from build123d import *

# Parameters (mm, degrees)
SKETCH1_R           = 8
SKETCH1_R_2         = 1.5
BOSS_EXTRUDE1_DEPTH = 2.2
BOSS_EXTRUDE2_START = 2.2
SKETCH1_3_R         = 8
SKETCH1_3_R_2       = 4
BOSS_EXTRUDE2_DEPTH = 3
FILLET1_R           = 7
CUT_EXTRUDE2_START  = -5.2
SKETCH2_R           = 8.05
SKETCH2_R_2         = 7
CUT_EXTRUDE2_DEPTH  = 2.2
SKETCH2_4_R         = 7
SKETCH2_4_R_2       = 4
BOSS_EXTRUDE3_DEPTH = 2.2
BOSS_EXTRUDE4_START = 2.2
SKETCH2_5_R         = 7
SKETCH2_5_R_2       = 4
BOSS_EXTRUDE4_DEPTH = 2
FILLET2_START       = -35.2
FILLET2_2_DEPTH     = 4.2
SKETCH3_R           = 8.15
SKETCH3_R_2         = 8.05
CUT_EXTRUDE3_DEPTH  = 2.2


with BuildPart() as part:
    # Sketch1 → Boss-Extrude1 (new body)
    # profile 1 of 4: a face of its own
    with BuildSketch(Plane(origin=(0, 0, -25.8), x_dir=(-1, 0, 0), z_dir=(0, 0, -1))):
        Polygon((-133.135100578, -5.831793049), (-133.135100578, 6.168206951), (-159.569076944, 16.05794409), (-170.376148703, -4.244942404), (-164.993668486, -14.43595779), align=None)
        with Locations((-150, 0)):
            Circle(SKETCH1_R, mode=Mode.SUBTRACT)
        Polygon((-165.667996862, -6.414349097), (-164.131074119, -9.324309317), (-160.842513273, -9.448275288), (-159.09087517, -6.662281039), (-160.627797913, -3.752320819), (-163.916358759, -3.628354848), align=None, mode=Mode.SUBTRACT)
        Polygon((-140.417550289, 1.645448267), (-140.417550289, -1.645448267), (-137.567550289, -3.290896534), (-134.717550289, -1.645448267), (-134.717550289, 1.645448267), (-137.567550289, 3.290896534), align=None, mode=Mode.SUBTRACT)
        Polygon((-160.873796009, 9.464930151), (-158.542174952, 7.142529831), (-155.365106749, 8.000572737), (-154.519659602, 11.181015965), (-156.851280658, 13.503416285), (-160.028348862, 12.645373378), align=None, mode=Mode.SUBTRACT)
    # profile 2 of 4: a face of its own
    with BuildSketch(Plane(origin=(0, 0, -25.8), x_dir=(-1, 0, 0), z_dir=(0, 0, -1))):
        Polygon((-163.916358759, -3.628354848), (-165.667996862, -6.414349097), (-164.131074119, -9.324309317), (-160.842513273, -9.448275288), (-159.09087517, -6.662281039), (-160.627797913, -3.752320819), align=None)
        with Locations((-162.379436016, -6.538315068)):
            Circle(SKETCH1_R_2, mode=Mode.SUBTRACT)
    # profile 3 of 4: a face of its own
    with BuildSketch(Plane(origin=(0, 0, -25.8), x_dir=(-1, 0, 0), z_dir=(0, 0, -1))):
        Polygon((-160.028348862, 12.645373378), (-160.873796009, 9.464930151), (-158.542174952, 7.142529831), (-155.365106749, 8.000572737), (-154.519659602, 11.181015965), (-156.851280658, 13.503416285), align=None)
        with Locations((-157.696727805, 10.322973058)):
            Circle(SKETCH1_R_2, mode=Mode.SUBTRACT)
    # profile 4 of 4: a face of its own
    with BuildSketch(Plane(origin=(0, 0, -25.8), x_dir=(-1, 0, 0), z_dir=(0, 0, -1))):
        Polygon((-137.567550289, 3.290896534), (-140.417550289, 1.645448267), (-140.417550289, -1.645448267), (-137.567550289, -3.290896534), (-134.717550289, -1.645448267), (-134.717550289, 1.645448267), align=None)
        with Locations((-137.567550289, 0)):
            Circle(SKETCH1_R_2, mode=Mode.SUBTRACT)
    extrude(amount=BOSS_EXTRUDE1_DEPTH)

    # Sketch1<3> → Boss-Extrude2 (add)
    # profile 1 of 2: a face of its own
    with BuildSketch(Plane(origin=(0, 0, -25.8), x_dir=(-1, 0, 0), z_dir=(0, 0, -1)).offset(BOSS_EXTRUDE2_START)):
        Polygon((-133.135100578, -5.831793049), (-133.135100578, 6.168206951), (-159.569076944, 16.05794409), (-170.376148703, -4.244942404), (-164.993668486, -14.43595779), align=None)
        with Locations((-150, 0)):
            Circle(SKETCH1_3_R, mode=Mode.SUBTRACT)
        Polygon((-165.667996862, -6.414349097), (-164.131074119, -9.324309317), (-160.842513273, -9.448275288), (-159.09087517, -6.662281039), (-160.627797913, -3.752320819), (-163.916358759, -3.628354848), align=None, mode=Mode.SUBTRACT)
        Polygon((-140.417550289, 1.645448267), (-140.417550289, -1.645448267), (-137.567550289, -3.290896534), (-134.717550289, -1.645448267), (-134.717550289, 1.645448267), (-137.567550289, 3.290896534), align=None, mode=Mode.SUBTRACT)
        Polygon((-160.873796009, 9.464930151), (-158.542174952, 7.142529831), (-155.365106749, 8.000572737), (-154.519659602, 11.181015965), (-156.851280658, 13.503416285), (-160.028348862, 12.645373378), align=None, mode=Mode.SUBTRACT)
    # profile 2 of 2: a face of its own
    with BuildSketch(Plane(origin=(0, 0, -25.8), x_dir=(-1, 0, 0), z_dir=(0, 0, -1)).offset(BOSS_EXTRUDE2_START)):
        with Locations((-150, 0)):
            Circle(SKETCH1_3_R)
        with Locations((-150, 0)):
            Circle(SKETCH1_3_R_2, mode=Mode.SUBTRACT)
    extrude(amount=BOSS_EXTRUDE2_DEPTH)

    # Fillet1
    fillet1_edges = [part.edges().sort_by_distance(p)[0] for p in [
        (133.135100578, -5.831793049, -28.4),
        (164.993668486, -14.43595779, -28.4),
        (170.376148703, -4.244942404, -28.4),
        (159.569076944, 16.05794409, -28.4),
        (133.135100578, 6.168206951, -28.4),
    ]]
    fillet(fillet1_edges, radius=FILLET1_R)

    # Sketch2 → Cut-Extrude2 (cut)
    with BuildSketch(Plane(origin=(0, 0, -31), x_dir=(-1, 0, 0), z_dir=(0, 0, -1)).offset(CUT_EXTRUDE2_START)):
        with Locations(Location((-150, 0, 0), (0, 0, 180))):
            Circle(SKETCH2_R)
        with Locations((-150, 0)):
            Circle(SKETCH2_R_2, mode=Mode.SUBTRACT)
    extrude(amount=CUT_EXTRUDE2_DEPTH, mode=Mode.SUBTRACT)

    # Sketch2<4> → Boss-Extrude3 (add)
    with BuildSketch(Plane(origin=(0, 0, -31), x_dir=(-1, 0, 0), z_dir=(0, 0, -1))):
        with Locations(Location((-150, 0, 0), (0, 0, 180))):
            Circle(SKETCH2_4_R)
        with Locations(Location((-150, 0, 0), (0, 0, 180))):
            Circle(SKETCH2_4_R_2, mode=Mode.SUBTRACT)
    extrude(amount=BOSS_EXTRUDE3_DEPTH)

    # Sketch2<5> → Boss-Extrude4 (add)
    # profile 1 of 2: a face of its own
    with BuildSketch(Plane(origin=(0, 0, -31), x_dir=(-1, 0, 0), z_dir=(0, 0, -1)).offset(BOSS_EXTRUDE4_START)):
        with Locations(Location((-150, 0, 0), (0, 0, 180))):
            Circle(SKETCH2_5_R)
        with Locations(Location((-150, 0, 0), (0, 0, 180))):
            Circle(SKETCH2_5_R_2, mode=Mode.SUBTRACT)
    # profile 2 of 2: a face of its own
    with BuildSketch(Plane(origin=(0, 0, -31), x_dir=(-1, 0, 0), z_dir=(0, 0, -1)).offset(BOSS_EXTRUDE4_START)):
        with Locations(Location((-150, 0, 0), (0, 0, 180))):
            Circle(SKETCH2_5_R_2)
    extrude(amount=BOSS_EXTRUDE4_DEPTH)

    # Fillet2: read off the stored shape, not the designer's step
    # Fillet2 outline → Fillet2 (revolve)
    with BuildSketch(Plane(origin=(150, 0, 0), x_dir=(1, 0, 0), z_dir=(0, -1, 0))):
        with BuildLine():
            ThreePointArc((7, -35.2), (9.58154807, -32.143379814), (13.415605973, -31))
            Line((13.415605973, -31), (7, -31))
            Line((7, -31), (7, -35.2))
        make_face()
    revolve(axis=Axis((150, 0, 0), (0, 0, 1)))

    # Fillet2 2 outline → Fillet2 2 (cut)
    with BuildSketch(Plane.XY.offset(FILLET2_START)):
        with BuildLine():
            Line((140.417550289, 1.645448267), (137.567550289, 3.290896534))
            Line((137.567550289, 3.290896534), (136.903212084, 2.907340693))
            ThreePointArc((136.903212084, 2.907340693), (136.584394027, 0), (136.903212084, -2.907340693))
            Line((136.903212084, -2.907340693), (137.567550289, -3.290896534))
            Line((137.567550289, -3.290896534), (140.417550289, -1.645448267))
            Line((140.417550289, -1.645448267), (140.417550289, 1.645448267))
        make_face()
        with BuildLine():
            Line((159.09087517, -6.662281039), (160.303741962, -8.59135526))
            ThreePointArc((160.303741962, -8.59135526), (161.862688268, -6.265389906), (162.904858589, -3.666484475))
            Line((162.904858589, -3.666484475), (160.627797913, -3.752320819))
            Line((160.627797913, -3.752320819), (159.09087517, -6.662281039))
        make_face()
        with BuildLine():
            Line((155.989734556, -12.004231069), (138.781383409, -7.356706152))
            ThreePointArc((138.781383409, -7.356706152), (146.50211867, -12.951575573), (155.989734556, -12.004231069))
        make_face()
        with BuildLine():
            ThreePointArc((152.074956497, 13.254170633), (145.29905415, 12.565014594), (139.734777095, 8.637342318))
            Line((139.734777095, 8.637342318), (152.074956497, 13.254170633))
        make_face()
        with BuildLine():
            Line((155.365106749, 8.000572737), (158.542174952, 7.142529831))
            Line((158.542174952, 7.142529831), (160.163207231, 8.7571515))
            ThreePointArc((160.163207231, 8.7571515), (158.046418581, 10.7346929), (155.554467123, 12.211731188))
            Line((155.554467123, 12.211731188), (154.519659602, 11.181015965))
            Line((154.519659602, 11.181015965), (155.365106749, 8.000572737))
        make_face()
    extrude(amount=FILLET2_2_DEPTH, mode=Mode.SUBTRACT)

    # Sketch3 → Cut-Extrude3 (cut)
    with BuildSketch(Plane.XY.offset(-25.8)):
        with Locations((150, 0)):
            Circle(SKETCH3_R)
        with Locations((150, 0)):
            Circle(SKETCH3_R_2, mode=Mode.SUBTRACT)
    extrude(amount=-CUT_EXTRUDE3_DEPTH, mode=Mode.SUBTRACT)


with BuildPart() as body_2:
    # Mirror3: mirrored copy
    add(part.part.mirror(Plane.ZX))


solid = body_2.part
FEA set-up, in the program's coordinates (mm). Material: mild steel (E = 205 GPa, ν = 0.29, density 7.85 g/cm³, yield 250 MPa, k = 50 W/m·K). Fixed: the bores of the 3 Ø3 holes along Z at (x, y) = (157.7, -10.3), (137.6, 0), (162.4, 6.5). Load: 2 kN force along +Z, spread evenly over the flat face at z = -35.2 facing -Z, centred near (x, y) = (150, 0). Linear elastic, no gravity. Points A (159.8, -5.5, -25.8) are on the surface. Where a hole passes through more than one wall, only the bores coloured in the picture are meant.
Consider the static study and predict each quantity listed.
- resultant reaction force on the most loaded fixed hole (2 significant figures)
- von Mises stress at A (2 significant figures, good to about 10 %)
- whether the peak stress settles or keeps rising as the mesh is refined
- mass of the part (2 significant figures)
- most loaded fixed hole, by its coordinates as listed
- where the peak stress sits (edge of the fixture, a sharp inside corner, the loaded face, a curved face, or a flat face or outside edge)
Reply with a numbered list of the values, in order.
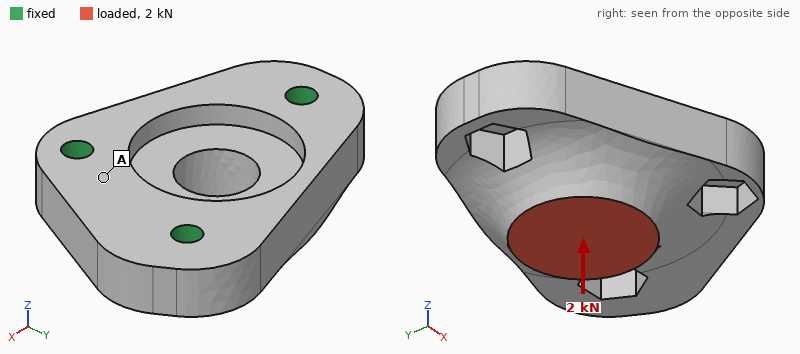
1. 1.1 kN
2. 16 MPa
3. keeps rising
4. 29 g
5. (137.6, 0)
6. edge of the fixture
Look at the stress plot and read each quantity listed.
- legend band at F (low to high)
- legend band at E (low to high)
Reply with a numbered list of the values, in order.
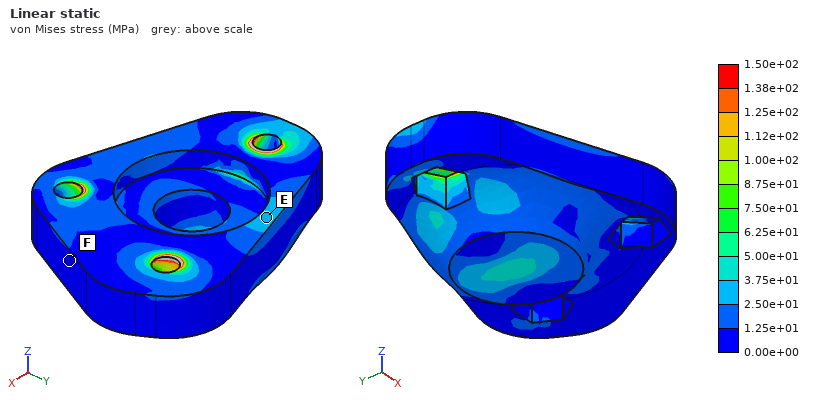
1. 0.00e+00 to 1.25e+01 MPa
2. 2.50e+01 to 3.75e+01 MPa
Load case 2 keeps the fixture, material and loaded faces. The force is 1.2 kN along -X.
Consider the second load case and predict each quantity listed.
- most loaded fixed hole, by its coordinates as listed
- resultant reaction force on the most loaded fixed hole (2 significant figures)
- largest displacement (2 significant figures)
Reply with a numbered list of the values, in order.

1. (137.6, 0)
2. 670 N
3. 1.9 µm
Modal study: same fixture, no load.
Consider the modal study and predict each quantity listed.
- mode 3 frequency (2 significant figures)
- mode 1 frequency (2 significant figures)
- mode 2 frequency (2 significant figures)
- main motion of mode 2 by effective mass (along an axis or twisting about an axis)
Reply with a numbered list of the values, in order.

1. 37 kHz
2. 25 kHz
3. 31 kHz
4. along Z
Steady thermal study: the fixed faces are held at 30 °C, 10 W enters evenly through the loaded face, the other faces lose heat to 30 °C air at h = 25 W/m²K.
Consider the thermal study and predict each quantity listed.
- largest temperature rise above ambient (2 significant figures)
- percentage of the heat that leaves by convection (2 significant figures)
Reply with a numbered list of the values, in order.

1. 20 K
2. 4.2 %
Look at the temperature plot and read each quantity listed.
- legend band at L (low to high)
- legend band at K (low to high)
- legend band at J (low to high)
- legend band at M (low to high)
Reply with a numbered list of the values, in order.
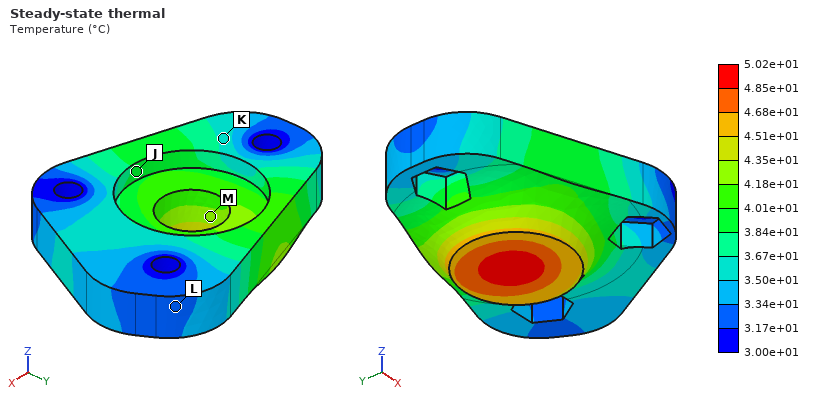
1. 3.17e+01 to 3.34e+01 °C
2. 3.50e+01 to 3.67e+01 °C
3. 3.84e+01 to 4.01e+01 °C
4. 4.18e+01 to 4.35e+01 °C
